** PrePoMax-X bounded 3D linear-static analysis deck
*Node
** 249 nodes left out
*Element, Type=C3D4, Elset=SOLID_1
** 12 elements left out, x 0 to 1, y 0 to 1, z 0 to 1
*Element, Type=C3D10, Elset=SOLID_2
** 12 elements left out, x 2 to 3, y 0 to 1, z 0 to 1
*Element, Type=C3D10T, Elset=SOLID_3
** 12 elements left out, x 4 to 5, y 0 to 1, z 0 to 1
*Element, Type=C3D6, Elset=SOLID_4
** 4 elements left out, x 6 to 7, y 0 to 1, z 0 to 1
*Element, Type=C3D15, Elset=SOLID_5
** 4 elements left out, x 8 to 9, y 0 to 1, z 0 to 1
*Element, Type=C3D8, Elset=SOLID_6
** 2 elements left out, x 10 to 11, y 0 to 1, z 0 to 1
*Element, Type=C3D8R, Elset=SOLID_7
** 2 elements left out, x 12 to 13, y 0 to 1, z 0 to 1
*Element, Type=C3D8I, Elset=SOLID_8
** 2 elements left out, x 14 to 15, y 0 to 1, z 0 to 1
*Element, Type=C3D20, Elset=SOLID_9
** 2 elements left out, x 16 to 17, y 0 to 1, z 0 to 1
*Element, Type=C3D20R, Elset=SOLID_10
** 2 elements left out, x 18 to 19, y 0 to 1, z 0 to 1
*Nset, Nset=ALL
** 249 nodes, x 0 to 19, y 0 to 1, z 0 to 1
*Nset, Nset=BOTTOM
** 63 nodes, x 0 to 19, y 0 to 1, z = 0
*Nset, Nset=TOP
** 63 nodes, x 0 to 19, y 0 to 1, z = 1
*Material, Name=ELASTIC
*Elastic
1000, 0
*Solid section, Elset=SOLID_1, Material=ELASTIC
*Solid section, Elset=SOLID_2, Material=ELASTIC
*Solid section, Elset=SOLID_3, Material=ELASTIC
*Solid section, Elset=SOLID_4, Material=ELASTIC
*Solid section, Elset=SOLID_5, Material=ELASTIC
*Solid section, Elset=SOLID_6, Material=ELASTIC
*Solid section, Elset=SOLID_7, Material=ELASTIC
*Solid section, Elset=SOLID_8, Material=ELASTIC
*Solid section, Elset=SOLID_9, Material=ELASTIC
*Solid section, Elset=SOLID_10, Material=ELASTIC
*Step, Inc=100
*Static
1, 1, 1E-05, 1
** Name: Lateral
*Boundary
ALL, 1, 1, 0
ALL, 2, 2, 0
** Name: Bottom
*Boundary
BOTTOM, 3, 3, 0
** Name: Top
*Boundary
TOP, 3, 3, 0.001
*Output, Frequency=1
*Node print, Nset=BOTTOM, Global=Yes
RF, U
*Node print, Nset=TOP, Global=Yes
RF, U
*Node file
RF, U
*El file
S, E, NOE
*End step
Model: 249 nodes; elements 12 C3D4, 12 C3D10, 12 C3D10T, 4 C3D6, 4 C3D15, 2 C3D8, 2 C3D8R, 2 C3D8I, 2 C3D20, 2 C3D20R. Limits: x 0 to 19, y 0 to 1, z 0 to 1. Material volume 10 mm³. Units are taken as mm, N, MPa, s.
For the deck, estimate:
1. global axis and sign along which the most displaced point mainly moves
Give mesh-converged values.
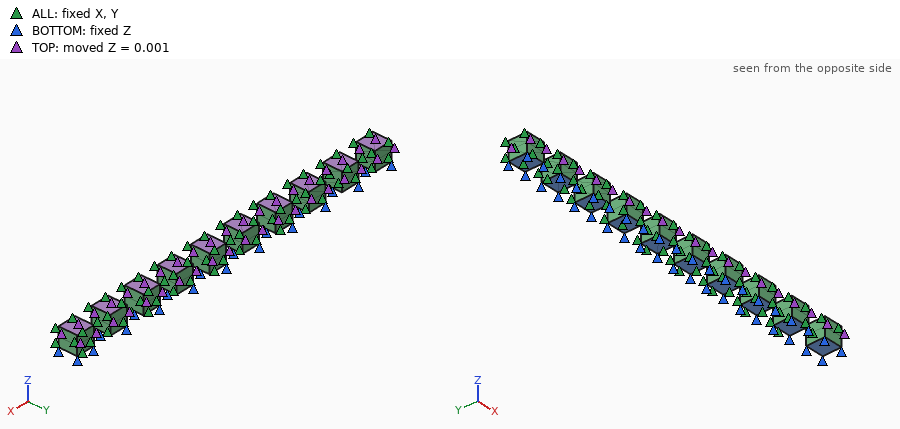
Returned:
+Z
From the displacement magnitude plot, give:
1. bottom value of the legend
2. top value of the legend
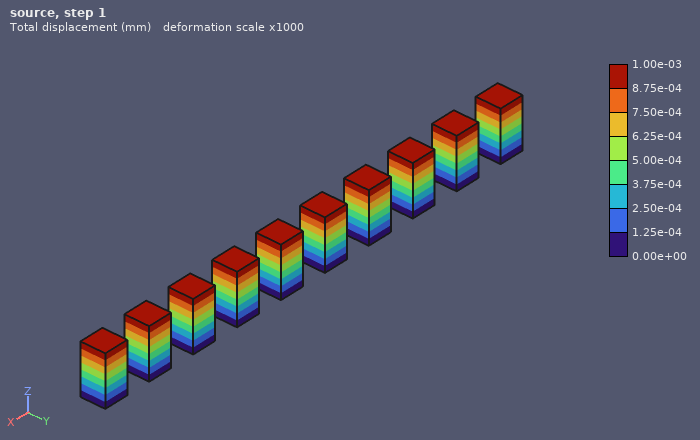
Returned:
0.00e+00 mm
1.00e-03 mm
